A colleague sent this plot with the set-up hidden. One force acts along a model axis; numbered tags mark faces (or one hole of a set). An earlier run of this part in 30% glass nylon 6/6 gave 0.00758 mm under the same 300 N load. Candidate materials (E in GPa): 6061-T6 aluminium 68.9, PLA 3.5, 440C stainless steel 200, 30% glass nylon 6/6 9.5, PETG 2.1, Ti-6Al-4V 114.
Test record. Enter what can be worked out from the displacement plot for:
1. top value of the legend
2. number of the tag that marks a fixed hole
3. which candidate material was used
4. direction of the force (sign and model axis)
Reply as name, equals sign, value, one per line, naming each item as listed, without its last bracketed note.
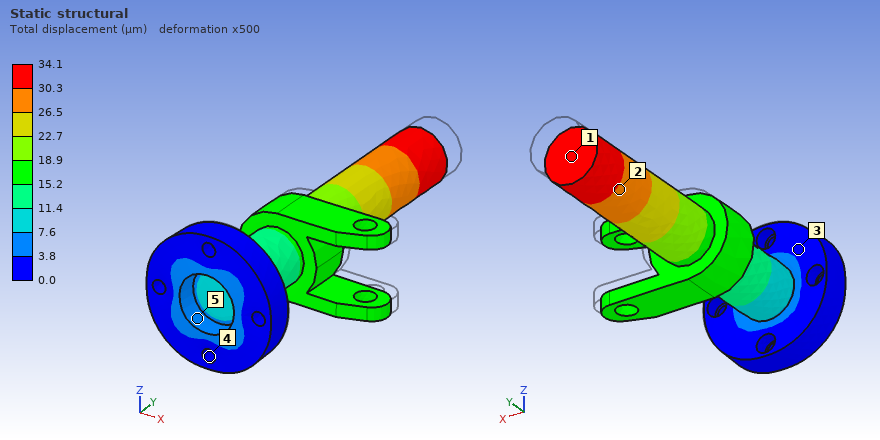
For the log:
top value of the legend = 34.1 µm
number of the tag that marks a fixed hole = 4
which candidate material was used = PETG
direction of the force = -Y
